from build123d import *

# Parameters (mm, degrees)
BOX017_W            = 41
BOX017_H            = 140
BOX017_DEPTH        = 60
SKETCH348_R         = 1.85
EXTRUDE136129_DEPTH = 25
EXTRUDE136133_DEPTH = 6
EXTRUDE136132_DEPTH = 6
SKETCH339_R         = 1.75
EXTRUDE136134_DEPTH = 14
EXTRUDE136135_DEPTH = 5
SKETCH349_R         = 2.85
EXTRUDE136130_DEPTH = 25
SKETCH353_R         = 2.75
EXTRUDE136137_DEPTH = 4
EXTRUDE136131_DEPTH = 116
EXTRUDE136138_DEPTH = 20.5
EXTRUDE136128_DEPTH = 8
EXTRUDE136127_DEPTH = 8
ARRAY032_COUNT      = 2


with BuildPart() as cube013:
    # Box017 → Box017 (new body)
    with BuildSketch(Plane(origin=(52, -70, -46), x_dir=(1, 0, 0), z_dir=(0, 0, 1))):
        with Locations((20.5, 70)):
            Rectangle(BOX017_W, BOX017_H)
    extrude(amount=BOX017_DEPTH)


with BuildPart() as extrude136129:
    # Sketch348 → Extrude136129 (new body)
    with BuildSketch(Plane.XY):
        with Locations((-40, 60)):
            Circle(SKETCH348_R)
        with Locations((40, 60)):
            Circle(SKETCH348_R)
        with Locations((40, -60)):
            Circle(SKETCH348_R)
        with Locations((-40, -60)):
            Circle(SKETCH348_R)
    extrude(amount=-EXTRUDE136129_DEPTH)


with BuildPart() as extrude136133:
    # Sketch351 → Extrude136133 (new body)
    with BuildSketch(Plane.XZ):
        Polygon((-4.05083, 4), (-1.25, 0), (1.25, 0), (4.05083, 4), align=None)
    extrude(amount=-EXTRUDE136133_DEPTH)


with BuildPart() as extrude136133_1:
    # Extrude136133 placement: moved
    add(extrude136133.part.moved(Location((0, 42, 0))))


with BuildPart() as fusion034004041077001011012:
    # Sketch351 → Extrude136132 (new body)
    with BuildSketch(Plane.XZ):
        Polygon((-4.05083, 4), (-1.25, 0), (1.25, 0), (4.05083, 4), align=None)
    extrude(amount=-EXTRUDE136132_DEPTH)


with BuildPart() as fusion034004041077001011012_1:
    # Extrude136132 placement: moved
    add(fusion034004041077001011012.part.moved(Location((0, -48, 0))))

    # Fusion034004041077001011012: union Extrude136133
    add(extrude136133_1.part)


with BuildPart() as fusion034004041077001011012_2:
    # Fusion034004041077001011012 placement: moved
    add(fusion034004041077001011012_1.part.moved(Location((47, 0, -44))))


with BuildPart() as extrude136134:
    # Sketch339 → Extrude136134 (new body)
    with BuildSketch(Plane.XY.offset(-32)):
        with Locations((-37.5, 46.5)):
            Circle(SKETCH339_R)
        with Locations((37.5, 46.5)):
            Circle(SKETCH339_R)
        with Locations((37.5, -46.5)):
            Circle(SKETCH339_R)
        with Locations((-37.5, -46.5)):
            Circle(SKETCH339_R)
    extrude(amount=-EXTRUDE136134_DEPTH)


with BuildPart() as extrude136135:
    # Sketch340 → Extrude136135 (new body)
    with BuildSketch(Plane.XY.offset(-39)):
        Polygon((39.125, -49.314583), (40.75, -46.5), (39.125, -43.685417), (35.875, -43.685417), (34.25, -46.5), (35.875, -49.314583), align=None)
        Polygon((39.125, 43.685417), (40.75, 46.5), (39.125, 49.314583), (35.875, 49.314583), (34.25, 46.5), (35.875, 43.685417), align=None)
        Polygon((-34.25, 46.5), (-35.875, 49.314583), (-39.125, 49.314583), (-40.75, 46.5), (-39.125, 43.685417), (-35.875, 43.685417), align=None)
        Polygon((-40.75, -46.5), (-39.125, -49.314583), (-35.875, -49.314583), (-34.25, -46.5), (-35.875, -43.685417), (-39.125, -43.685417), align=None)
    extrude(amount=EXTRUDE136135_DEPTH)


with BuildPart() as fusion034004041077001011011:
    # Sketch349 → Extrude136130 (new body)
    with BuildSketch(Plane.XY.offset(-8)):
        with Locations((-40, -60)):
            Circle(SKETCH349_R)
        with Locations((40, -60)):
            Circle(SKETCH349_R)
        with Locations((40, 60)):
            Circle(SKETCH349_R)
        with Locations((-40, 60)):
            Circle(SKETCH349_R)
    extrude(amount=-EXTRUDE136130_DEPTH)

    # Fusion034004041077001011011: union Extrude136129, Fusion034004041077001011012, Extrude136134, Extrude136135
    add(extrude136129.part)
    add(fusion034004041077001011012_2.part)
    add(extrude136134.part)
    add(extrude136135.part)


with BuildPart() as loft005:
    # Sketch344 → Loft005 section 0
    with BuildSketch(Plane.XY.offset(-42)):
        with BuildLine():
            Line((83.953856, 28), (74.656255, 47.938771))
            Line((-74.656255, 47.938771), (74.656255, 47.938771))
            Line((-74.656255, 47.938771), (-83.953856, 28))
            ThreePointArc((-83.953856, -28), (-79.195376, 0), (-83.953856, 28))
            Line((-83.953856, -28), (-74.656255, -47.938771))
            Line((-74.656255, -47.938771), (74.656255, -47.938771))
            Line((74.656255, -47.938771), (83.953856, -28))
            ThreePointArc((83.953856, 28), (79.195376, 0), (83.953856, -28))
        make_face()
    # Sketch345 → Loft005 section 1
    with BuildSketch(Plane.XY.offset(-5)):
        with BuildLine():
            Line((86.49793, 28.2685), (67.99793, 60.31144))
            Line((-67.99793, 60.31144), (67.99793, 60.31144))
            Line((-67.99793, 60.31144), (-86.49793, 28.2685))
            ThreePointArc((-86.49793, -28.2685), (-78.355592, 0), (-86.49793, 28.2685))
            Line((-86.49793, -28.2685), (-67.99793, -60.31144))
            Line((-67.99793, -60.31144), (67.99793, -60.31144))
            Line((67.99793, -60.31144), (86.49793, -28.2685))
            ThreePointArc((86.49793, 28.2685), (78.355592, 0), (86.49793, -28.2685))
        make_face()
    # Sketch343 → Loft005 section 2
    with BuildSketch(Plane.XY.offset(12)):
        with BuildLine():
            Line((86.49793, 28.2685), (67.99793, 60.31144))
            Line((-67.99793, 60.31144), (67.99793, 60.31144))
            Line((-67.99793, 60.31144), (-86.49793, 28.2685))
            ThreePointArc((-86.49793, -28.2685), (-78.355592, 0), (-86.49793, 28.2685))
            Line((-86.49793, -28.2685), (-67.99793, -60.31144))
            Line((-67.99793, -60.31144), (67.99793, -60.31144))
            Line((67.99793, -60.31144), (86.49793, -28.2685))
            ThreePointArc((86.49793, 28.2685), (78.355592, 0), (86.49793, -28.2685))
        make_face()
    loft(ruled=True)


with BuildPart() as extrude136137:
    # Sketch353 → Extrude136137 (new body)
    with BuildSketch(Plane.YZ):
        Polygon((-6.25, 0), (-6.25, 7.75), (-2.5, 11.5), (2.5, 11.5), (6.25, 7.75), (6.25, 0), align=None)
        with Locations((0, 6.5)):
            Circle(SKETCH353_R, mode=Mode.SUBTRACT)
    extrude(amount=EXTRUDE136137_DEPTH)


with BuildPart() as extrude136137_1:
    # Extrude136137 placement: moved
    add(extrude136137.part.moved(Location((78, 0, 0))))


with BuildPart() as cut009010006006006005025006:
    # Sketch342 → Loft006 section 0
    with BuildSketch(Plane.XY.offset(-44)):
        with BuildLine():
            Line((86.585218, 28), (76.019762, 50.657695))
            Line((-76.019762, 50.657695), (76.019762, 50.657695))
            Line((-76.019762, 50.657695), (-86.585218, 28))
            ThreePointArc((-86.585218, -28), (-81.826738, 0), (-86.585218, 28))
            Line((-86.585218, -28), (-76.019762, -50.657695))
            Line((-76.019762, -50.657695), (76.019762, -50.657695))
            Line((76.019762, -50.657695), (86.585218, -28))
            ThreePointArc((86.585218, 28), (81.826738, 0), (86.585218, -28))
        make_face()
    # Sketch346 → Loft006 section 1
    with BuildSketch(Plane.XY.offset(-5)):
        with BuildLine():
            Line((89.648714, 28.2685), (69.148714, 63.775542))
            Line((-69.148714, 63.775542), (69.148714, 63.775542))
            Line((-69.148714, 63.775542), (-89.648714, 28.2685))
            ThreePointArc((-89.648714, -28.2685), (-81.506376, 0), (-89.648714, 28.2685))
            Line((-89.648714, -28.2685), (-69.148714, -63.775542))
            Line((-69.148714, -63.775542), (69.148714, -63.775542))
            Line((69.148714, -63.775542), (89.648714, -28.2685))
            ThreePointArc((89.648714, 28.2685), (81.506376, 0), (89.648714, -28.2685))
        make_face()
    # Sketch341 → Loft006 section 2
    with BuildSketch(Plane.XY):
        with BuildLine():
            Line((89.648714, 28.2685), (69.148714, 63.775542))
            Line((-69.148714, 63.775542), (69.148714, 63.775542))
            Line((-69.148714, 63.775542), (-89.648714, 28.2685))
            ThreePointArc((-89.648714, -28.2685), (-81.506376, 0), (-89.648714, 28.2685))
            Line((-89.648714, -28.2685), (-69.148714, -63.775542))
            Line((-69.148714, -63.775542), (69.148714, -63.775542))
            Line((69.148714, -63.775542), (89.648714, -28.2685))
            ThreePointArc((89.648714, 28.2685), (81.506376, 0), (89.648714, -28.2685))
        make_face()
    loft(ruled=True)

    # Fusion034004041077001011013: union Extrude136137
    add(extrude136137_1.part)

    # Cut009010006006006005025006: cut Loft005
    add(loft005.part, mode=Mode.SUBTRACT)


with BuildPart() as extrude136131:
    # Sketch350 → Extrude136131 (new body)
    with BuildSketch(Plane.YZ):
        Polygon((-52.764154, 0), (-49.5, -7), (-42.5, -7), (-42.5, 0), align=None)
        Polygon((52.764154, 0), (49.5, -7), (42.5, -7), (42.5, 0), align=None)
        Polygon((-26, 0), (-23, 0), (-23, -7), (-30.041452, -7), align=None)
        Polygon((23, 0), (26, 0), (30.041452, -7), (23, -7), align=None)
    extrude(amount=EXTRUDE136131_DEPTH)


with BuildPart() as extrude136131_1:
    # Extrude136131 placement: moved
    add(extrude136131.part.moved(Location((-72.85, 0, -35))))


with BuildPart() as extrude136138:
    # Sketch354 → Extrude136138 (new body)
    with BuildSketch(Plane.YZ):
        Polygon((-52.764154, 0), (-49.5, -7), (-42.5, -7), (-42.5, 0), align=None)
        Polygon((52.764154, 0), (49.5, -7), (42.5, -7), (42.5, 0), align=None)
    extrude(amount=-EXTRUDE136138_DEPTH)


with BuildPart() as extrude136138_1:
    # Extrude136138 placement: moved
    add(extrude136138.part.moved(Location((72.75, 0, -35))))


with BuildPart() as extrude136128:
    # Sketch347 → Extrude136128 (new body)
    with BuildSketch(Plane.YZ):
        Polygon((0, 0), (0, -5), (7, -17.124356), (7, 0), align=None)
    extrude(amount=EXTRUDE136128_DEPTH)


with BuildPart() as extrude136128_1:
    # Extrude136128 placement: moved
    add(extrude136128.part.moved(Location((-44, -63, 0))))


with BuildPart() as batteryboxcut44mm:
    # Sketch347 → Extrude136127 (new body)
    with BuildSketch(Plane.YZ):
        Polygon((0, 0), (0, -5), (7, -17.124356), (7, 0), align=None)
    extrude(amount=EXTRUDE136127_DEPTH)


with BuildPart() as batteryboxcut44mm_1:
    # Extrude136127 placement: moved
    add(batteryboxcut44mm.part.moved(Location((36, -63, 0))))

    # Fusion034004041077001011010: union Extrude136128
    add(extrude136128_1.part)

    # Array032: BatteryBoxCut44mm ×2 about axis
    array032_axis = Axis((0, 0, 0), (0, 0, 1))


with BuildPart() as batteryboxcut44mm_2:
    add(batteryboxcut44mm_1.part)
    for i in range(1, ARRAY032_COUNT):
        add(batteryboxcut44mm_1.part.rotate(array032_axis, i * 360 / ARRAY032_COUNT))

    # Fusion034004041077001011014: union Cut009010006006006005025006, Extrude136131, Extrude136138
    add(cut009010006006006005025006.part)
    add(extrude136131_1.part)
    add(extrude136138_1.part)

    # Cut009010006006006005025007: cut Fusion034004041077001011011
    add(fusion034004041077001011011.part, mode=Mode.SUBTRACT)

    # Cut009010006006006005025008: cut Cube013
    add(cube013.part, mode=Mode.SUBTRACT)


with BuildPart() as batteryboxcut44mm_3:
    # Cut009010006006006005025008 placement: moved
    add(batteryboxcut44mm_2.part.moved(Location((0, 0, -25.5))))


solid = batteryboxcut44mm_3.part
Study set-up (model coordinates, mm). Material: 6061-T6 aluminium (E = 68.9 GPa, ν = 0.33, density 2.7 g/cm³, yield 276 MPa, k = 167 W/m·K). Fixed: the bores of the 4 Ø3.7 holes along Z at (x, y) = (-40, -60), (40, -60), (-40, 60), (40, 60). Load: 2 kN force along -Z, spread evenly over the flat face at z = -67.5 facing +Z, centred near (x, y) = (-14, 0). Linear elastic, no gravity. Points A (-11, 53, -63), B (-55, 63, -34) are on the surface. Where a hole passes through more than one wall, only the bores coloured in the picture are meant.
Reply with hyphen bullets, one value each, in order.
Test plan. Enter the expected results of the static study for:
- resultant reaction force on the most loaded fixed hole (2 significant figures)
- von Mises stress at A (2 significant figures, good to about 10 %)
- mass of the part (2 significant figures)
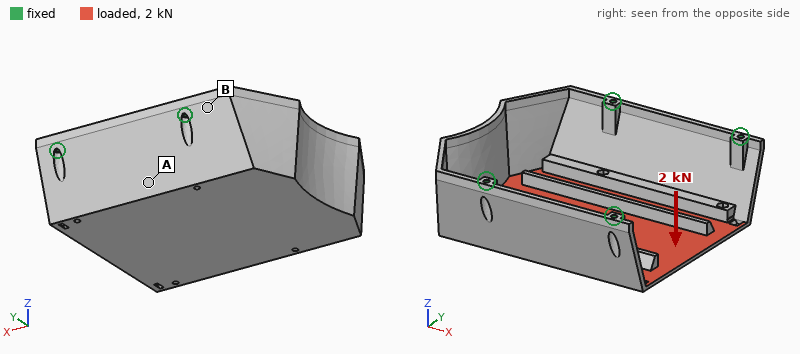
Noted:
- 800 N
- 20 MPa
- 260 g
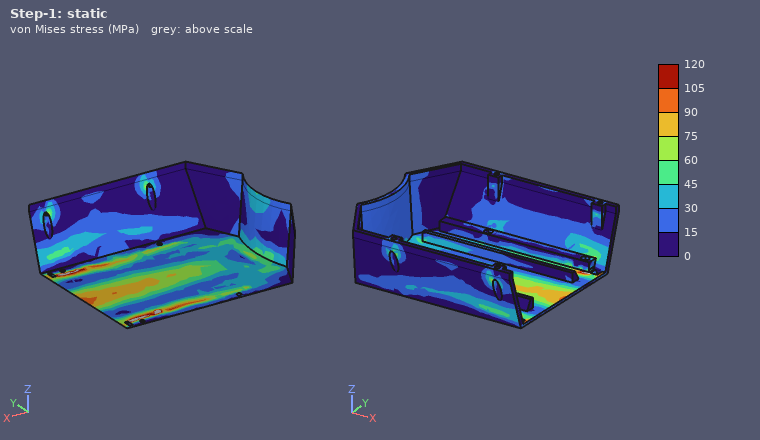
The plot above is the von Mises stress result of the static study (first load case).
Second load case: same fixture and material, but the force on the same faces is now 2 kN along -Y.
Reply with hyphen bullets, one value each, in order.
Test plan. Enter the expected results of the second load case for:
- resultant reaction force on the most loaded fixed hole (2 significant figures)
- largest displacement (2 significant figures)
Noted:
- 1000 N
- 0.35 mm
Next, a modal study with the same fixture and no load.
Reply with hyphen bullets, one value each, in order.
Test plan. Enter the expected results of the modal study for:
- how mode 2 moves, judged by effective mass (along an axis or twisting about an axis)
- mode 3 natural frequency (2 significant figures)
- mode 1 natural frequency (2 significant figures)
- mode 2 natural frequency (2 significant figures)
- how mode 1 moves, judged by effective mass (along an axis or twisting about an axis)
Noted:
- along Z
- 1700 Hz
- 950 Hz
- 1300 Hz
- along Y
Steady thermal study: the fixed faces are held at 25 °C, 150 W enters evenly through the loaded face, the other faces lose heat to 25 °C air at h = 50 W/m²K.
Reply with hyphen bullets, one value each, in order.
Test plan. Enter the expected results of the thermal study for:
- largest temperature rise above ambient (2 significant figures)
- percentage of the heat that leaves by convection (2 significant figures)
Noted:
- 60 K
- 55 %
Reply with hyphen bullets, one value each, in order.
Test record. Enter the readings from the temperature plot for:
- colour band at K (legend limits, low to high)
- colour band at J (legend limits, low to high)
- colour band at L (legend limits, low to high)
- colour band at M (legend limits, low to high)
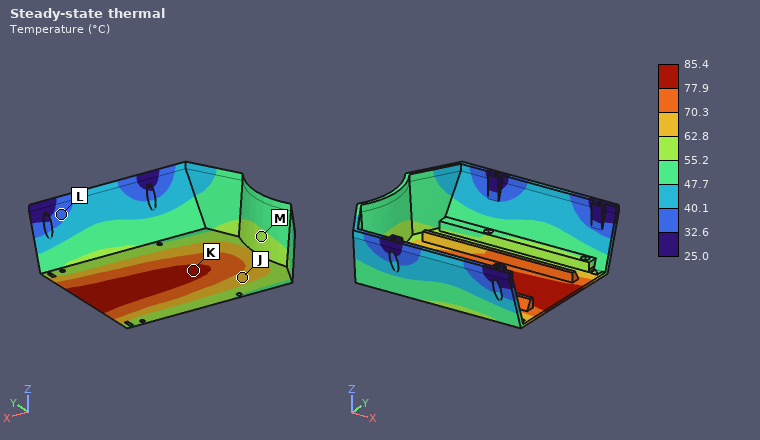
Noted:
- 77.9 to 85.4 °C
- 62.8 to 70.3 °C
- 32.6 to 40.1 °C
- 55.2 to 62.8 °C
